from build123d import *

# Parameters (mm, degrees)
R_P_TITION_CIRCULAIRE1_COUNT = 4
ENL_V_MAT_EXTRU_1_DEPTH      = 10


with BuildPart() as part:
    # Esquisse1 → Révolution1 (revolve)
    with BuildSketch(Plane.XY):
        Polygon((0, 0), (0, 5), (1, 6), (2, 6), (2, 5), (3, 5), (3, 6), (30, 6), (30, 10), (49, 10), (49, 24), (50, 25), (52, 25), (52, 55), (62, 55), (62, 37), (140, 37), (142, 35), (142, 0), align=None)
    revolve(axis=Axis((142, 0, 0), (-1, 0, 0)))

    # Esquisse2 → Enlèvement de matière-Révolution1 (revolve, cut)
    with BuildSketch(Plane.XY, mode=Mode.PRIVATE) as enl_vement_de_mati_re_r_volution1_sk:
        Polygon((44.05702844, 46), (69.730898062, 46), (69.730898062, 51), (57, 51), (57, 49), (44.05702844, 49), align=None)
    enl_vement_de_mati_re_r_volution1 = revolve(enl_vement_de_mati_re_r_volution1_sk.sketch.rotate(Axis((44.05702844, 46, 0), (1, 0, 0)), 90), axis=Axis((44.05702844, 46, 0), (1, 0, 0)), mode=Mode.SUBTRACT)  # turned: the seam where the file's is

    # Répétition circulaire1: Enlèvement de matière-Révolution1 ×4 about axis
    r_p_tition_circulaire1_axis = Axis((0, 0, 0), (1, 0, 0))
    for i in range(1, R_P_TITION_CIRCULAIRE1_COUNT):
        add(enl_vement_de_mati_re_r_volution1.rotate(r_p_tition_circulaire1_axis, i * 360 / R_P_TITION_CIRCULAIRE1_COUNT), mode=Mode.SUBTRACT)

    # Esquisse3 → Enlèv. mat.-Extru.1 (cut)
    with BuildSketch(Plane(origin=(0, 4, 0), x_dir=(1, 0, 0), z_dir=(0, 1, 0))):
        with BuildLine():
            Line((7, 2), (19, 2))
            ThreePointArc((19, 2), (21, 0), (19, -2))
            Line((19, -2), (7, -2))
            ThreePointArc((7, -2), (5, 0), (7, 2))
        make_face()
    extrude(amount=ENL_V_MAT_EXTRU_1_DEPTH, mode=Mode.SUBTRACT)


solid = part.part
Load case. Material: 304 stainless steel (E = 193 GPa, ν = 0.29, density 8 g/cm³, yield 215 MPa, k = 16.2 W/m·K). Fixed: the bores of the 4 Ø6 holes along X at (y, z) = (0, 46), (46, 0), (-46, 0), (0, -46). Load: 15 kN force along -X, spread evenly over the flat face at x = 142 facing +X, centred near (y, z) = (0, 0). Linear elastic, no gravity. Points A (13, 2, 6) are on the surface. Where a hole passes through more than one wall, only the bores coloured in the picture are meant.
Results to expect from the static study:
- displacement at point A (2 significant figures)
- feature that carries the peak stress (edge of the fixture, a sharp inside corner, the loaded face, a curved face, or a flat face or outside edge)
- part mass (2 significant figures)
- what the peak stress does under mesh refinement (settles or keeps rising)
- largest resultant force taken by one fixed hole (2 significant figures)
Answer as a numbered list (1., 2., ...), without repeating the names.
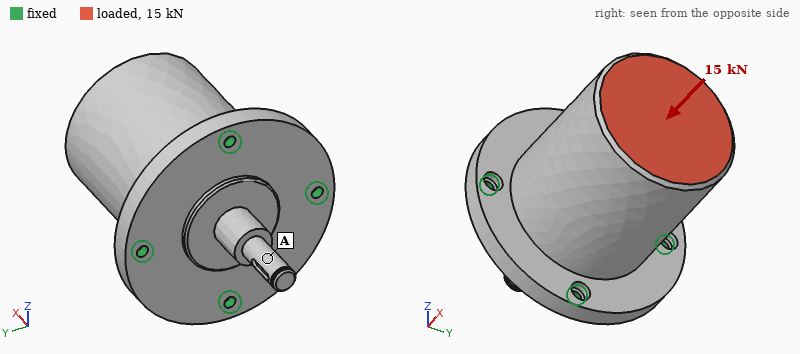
1. 7.3 µm
2. edge of the fixture
3. 3.6 kg
4. keeps rising
5. 4.3 kN
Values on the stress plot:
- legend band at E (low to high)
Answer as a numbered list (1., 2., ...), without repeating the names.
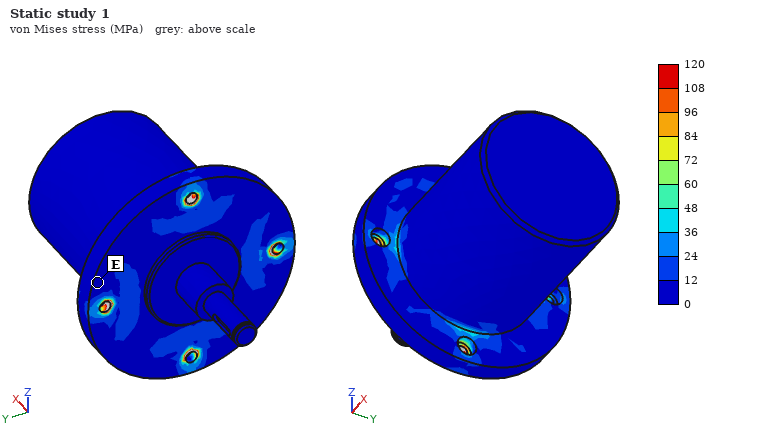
1. 0 to 12 MPa
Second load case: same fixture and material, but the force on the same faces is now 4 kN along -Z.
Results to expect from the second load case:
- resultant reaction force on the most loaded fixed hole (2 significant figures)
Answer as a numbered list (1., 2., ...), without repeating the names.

1. 4.5 kN
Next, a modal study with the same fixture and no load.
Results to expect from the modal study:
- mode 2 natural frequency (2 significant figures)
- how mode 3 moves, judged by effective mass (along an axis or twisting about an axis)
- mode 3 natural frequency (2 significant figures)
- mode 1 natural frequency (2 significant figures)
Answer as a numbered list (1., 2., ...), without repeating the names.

1. 2300 Hz
2. along X
3. 3900 Hz
4. 2300 Hz
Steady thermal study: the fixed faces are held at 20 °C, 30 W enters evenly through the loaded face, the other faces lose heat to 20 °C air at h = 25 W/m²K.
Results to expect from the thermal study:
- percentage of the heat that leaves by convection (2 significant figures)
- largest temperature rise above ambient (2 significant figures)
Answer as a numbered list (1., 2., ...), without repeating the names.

1. 57 %
2. 42 K
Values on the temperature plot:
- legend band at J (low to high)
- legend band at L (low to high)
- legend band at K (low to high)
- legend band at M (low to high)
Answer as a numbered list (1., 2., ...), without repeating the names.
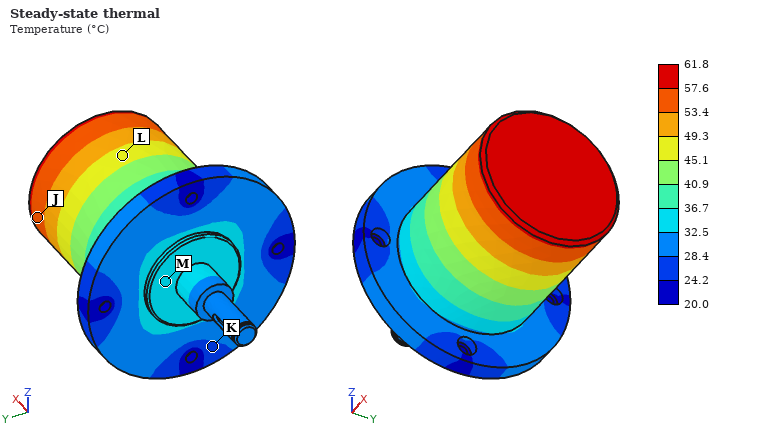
1. 53.4 to 57.6 °C
2. 45.1 to 49.3 °C
3. 24.2 to 28.4 °C
4. 32.5 to 36.7 °C
